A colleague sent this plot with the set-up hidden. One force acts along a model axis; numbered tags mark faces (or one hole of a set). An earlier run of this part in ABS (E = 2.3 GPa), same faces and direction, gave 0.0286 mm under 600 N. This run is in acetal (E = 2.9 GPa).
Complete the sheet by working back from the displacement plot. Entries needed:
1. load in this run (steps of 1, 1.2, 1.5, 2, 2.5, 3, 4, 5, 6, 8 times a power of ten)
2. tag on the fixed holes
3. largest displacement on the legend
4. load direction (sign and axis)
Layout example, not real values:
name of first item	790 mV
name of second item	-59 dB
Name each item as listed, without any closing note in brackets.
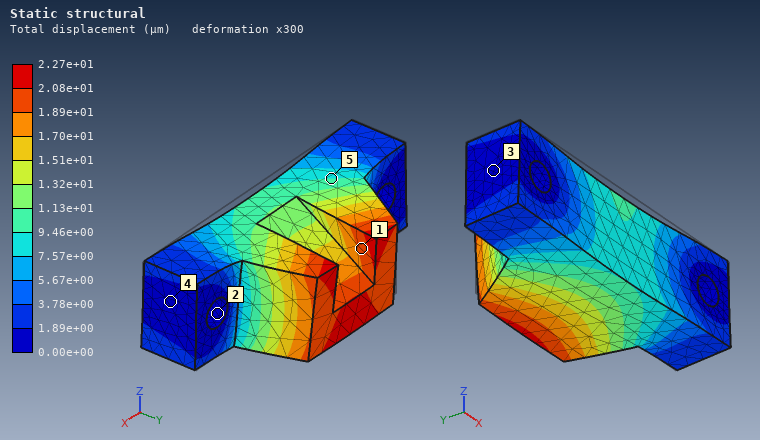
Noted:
load in this run	600 N
tag on the fixed holes	2
largest displacement on the legend	2.27e+01 µm
load direction	-Z
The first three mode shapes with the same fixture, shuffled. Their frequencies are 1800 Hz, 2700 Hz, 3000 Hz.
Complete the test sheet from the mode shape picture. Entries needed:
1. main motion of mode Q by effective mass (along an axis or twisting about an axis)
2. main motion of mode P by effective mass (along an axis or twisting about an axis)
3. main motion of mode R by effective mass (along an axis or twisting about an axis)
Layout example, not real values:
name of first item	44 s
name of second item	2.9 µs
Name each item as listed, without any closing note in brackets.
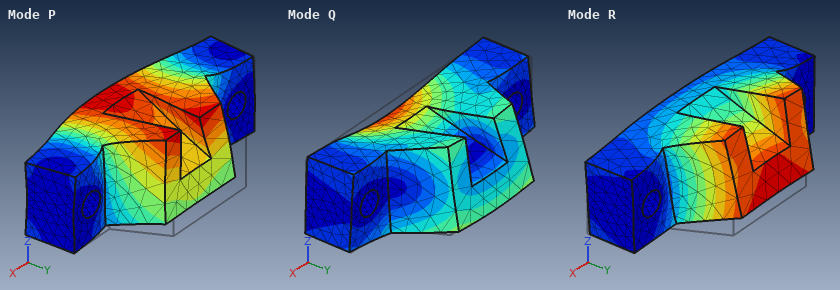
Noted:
main motion of mode Q by effective mass	along Z
main motion of mode P by effective mass	along Y
main motion of mode R by effective mass	along Z
